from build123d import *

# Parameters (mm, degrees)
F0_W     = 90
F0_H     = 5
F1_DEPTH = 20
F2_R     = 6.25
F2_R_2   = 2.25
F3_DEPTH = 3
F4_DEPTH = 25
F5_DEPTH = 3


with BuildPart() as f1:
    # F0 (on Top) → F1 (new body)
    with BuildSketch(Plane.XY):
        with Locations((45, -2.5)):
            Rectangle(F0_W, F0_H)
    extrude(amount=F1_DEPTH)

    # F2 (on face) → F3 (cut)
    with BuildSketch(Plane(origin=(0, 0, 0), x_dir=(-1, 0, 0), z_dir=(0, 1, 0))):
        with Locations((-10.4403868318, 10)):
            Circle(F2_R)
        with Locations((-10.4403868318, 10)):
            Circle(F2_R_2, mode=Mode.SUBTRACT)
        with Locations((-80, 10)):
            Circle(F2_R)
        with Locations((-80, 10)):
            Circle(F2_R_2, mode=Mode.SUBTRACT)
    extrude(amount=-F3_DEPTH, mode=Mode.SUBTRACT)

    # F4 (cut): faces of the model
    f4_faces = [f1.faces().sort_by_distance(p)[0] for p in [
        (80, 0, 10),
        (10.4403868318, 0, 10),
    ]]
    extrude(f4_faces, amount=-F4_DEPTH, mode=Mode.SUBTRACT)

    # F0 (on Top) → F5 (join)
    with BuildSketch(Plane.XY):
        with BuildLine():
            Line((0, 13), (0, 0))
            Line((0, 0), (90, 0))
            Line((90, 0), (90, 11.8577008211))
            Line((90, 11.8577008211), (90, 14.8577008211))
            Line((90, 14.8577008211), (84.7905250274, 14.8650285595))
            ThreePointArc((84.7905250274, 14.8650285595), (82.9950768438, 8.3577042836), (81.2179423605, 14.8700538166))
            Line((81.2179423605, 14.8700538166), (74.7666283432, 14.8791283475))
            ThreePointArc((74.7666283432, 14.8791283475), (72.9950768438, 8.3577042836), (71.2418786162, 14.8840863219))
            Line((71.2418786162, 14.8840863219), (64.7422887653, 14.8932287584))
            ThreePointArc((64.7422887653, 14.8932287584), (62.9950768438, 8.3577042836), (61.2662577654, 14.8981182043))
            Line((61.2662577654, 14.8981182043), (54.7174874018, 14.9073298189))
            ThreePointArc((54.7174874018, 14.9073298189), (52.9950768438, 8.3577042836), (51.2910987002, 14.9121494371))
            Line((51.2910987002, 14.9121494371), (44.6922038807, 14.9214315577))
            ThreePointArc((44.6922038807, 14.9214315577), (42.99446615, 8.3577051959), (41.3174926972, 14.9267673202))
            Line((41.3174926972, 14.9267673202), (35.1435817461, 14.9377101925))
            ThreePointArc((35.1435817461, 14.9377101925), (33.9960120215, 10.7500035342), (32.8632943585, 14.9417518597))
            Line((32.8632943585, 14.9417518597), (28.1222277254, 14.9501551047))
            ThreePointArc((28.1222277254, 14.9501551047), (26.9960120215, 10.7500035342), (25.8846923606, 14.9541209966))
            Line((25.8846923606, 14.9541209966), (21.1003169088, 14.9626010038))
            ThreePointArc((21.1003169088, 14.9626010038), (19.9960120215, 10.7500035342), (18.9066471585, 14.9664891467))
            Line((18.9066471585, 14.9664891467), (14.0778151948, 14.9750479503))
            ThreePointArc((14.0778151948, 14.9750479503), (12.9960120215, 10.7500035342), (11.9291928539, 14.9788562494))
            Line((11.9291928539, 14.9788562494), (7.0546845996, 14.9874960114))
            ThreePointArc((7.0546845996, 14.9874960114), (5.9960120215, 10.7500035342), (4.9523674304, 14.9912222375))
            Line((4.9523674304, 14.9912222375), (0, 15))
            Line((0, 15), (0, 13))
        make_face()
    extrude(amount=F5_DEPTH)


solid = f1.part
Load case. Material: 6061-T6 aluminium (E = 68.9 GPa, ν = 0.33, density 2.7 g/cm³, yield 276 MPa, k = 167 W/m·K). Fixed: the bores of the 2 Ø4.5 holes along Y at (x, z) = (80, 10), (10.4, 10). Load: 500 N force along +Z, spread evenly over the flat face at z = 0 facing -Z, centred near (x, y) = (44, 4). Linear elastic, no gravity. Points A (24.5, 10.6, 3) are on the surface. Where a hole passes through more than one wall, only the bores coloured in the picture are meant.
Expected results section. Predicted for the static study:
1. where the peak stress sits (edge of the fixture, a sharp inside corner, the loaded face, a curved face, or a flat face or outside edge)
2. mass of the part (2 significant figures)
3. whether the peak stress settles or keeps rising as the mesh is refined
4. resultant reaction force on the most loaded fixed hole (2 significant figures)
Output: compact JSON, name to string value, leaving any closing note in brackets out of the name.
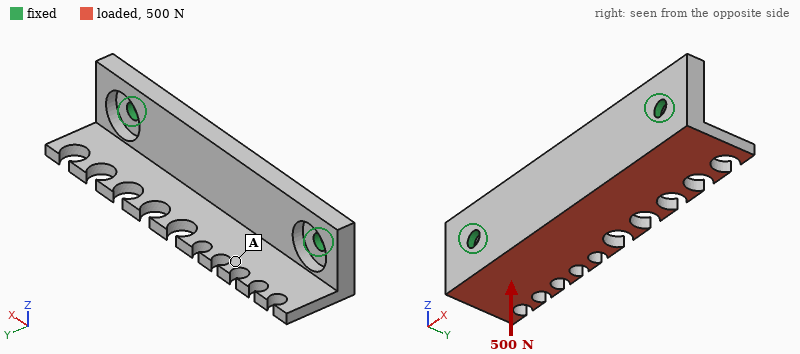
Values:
{"where the peak stress sits": "edge of the fixture", "mass of the part": "31 g", "whether the peak stress settles or keeps rising as the mesh is refined": "keeps rising", "resultant reaction force on the most loaded fixed hole": "260 N"}
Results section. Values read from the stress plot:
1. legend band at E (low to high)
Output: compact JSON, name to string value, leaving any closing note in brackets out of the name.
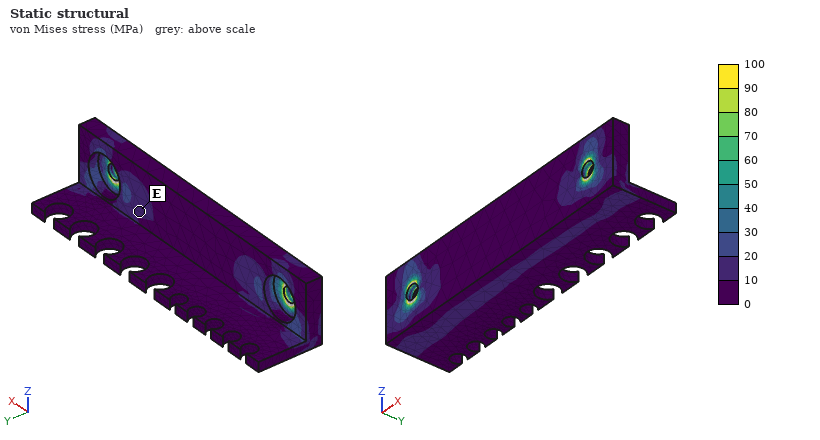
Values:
{"legend band at E": "10 to 20 MPa"}
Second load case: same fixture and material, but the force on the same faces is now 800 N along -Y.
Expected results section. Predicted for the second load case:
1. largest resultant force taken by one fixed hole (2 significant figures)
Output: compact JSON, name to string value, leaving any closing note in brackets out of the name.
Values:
{"largest resultant force taken by one fixed hole": "500 N"}
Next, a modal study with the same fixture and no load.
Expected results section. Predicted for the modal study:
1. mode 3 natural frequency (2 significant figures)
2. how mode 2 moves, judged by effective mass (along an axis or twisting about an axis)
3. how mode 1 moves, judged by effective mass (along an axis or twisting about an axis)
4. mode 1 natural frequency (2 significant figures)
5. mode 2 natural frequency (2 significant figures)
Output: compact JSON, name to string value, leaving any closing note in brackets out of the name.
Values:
{"mode 3 natural frequency": "6300 Hz", "how mode 2 moves, judged by effective mass": "along Y", "how mode 1 moves, judged by effective mass": "along Z", "mode 1 natural frequency": "3600 Hz", "mode 2 natural frequency": "5100 Hz"}
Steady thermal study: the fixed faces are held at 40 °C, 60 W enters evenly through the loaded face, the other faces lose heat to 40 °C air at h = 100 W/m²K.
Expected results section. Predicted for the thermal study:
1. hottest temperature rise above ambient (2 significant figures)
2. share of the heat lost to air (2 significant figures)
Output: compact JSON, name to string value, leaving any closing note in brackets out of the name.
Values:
{"hottest temperature rise above ambient": "35 K", "share of the heat lost to air": "21 %"}
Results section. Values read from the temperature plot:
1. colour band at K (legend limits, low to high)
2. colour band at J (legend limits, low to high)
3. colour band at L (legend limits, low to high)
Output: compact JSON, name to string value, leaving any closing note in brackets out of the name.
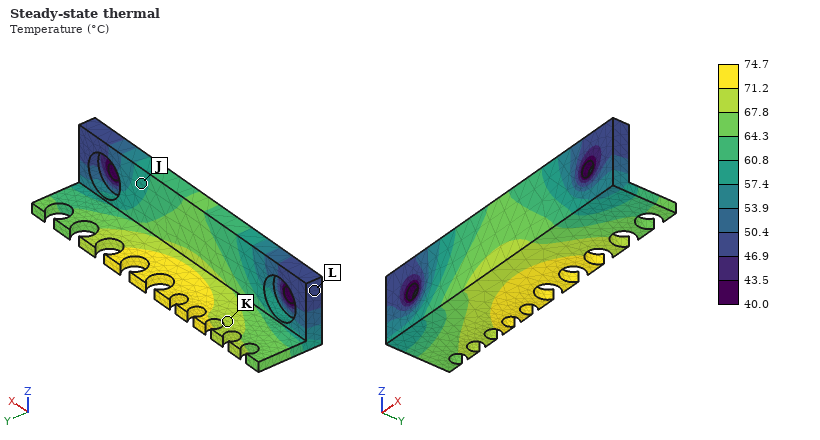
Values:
{"colour band at K": "67.8 to 71.2 °C", "colour band at J": "57.4 to 60.8 °C", "colour band at L": "46.9 to 50.4 °C"}
